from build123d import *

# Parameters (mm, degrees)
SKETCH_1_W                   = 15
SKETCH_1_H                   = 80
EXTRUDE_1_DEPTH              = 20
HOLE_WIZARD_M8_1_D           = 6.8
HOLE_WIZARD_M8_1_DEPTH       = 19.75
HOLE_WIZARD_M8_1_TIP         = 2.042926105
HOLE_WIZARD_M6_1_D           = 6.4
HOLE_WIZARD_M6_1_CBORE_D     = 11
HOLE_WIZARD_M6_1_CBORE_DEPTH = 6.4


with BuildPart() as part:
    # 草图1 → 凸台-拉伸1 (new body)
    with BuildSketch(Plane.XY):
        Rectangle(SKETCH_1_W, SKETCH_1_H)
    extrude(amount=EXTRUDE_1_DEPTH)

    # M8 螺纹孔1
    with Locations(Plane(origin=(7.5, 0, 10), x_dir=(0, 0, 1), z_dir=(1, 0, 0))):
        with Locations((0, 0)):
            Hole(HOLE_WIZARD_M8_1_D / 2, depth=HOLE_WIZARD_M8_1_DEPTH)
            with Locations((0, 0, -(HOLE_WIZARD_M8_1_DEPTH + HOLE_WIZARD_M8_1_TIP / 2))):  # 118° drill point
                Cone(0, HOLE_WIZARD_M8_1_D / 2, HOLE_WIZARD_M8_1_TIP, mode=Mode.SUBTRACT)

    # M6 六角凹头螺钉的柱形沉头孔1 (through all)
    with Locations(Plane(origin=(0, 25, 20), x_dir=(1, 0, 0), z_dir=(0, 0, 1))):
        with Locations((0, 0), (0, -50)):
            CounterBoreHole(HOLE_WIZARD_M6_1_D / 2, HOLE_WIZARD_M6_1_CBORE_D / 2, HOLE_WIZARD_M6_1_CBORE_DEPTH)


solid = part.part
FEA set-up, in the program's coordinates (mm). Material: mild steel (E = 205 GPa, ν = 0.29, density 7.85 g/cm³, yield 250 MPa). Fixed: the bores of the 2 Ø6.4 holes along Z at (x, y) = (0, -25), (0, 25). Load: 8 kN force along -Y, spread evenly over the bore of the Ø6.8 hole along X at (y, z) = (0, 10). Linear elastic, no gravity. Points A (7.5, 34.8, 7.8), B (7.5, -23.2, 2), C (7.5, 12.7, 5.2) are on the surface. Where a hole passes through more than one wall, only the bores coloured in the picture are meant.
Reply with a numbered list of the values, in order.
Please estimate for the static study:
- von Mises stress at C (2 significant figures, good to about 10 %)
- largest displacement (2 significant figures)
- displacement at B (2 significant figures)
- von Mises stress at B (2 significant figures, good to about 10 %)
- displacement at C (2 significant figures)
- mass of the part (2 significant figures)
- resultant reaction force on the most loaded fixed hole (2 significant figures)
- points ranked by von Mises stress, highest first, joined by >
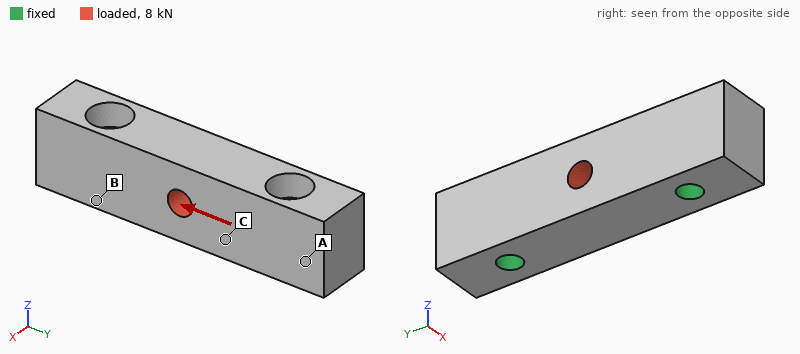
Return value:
1. 16 MPa
2. 2.3 µm
3. 0.34 µm
4. 8.3 MPa
5. 0.93 µm
6. 170 g
7. 4.0 kN
8. C > B > A
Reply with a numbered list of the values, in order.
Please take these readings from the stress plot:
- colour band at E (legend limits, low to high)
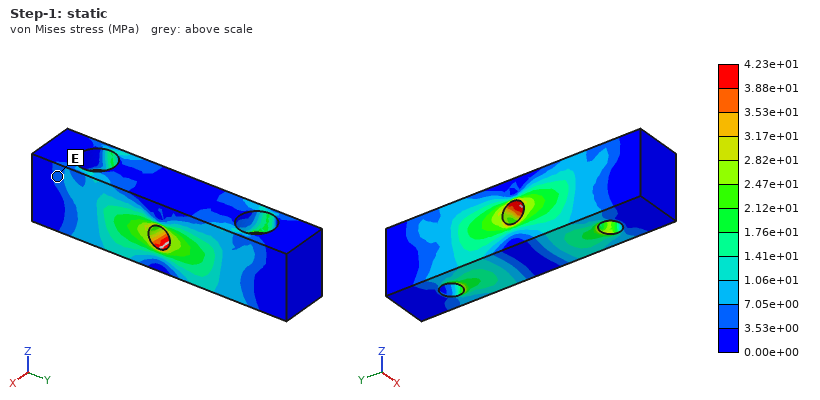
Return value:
1. 3.53e+00 to 7.05e+00 MPa
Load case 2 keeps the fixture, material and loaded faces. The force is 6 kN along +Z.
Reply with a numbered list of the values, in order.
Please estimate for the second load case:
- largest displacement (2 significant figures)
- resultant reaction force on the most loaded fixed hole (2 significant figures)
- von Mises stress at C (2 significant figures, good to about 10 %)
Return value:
1. 6.2 µm
2. 3.2 kN
3. 23 MPa
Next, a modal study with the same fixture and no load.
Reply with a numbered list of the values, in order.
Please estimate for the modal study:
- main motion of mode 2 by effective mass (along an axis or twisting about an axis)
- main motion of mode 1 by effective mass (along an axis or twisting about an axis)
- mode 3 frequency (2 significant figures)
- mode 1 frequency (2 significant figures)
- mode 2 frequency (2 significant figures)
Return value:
1. along Z
2. along X
3. 25 kHz
4. 18 kHz
5. 23 kHz
